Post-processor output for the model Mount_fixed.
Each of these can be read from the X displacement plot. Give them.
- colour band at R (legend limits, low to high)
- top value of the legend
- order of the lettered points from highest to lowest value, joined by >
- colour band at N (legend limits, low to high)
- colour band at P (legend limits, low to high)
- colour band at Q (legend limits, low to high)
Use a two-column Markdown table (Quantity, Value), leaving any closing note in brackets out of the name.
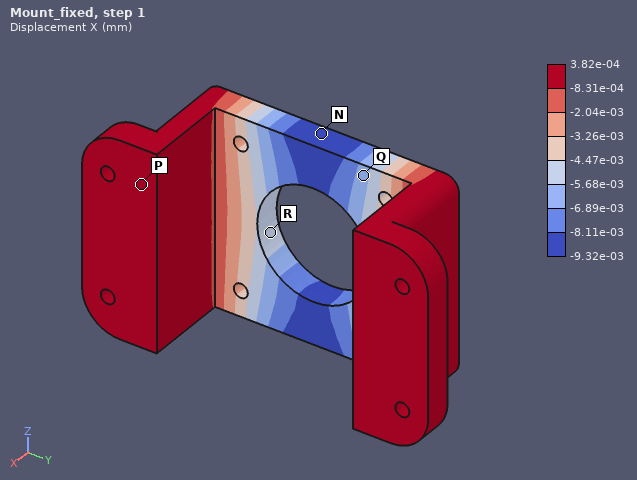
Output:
| Quantity | Value |
|---|---|
| colour band at R | -5.68e-03 to -4.47e-03 mm |
| top value of the legend | 3.82e-04 mm |
| order of the lettered points from highest to lowest value, joined by > | P > R > Q > N |
| colour band at N | -9.32e-03 to -8.11e-03 mm |
| colour band at P | -8.31e-04 to 3.82e-04 mm |
| colour band at Q | -6.89e-03 to -5.68e-03 mm |
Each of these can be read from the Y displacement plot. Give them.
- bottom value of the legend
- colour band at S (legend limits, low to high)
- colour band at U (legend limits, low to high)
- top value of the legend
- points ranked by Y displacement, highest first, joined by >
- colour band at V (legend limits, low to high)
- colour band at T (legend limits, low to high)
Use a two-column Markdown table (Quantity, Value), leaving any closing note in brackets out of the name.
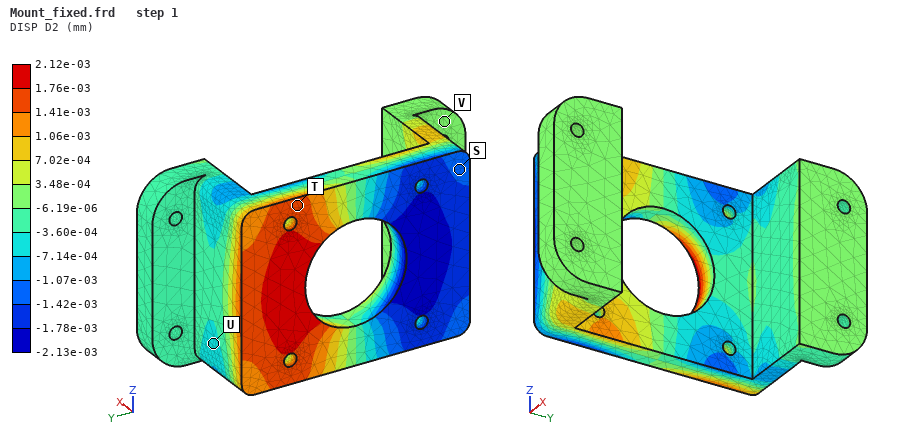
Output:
| Quantity | Value |
|---|---|
| bottom value of the legend | -2.13e-03 mm |
| colour band at S | -1.42e-03 to -1.07e-03 mm |
| colour band at U | -7.14e-04 to -3.60e-04 mm |
| top value of the legend | 2.12e-03 mm |
| points ranked by Y displacement, highest first, joined by > | T > V > U > S |
| colour band at V | -6.19e-06 to 3.48e-04 mm |
| colour band at T | 1.41e-03 to 1.76e-03 mm |
